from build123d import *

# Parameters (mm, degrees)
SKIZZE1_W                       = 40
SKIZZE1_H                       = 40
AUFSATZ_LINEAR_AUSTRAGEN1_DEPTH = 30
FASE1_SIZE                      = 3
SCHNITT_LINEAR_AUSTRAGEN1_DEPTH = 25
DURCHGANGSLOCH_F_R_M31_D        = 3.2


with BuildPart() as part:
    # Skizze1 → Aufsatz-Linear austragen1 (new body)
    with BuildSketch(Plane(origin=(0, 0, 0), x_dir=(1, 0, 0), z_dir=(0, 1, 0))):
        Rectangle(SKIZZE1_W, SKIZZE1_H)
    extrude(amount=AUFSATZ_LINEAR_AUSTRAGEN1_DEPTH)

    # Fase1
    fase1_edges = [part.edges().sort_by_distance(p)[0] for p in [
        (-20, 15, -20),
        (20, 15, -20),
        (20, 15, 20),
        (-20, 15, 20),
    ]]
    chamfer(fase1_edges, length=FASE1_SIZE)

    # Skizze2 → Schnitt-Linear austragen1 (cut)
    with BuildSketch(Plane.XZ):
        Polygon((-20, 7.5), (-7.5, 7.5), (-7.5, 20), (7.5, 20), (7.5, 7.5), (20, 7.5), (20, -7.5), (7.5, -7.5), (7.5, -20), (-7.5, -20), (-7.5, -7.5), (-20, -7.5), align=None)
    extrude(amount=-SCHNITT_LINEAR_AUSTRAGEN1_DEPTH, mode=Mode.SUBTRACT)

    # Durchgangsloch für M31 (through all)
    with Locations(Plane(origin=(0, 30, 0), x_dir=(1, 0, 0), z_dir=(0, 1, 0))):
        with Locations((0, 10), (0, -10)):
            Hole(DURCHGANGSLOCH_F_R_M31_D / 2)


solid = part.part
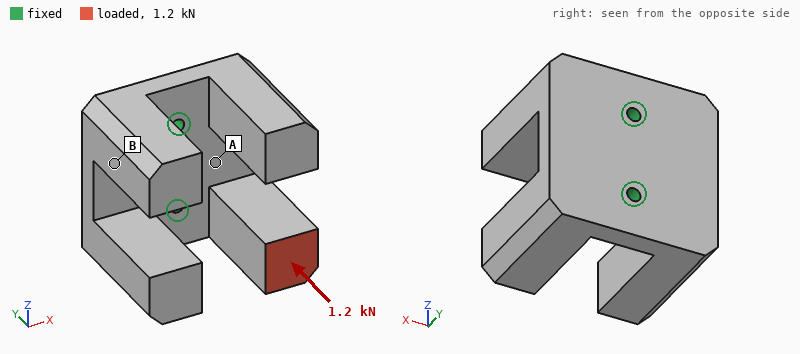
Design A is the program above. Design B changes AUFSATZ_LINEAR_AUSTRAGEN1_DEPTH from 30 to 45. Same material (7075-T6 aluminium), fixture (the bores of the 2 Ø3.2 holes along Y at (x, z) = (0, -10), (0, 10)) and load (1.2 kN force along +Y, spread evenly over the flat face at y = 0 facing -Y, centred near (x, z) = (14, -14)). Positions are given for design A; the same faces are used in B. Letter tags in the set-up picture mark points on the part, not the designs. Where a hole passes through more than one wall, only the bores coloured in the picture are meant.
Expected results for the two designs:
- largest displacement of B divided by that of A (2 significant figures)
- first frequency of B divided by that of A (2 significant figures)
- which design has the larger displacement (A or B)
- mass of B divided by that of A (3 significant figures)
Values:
0.057
3.2
A
2.02
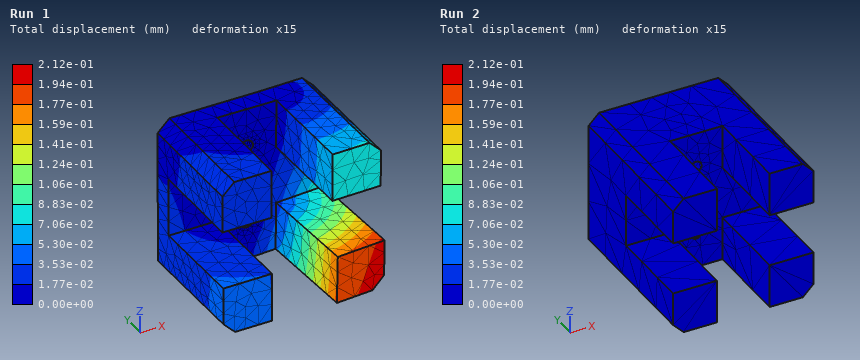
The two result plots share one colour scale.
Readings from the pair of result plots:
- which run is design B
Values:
Run 2
